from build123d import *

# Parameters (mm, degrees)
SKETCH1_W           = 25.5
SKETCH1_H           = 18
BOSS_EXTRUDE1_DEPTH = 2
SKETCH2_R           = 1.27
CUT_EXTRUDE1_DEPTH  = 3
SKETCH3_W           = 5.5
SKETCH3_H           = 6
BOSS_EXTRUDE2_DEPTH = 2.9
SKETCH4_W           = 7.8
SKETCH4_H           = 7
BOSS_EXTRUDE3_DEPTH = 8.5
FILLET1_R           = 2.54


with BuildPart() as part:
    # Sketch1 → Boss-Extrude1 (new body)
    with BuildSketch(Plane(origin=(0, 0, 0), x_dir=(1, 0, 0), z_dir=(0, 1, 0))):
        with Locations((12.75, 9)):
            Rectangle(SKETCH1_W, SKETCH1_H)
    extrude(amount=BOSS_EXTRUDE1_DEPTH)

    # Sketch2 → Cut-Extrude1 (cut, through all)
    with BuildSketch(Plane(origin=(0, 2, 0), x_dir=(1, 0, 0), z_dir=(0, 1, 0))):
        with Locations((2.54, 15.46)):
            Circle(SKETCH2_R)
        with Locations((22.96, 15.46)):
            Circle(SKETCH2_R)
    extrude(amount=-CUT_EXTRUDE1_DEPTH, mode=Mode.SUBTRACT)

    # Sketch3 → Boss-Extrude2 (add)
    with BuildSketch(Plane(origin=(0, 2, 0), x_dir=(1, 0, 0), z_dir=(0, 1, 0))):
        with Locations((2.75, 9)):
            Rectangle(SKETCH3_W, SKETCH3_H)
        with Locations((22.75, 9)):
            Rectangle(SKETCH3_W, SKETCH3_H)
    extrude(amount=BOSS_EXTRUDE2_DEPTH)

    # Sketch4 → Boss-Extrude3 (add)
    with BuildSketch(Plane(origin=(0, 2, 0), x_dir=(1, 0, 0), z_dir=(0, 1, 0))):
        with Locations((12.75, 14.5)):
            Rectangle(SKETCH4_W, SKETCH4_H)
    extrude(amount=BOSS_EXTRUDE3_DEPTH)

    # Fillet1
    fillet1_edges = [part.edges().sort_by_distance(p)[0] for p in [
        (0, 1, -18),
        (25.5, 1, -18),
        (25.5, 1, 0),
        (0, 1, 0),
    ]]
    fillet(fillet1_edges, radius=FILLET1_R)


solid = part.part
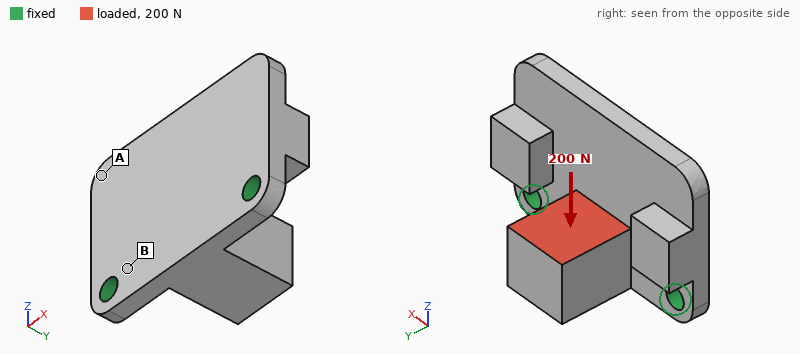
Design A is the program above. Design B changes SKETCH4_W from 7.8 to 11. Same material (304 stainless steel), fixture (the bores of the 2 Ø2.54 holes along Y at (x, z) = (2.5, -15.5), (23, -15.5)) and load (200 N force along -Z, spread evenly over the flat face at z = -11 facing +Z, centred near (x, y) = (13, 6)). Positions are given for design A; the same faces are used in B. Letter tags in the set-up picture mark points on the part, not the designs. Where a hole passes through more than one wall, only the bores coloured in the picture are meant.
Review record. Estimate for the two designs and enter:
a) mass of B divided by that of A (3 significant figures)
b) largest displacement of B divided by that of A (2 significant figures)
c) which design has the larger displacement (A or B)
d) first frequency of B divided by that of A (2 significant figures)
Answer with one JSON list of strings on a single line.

["1.12", "0.89", "A", "1.0"]
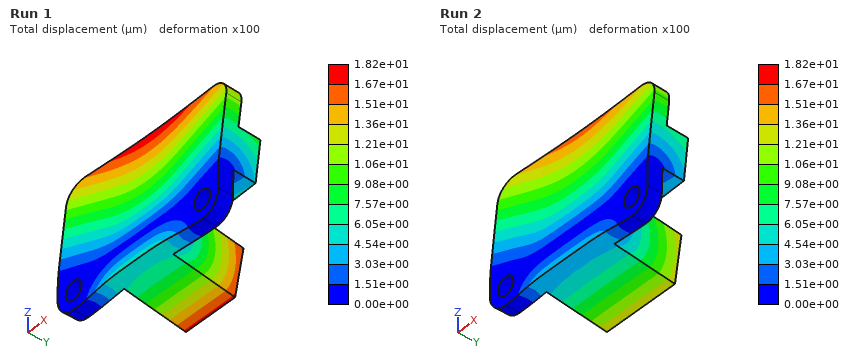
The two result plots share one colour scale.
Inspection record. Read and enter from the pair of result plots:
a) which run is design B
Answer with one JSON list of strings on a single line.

["Run 2"]
